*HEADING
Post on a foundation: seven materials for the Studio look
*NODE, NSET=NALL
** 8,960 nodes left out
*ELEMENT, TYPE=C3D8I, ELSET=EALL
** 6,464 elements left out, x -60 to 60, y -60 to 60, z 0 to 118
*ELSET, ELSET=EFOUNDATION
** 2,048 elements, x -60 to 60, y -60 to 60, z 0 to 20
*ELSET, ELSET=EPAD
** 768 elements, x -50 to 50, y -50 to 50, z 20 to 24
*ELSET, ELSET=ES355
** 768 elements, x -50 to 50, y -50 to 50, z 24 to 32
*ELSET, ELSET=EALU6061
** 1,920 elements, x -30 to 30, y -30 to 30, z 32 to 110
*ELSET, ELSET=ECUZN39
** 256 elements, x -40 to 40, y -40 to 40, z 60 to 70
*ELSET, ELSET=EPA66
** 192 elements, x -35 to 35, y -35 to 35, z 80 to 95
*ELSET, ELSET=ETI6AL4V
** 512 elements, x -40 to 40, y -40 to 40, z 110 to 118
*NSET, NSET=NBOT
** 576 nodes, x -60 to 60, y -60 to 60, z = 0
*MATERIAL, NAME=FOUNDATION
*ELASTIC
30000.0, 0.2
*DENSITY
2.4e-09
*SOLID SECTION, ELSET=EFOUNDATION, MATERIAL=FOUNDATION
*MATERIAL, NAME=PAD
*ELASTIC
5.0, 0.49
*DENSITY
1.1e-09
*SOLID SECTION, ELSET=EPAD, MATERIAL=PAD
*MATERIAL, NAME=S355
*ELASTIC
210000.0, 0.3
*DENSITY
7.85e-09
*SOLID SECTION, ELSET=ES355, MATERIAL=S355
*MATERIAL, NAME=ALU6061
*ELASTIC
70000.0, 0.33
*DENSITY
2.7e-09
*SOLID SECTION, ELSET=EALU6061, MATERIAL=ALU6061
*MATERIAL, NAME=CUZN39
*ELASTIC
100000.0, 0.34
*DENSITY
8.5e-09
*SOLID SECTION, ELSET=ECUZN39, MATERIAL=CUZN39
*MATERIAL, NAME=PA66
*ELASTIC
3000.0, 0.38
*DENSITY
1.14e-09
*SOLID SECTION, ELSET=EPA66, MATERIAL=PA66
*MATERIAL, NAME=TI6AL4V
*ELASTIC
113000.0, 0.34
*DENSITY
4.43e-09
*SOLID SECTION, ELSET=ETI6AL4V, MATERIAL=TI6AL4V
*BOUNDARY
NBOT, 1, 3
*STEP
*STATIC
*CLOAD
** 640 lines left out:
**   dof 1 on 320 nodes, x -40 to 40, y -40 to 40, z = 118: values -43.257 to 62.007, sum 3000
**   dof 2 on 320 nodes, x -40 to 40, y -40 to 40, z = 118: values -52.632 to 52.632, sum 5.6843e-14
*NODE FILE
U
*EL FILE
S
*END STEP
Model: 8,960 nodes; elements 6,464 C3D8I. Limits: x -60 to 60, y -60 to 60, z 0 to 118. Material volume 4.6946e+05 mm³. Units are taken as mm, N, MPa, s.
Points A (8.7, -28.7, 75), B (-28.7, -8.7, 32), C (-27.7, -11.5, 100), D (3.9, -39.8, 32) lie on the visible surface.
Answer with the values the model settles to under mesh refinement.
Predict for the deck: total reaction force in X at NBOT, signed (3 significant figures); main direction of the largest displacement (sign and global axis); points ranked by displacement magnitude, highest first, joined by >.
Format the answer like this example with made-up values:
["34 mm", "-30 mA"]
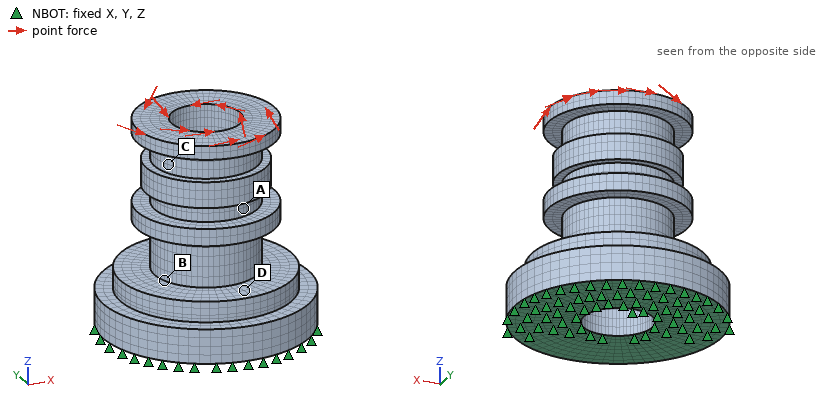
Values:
["-3000 N", "+X", "D > A > C > B"]
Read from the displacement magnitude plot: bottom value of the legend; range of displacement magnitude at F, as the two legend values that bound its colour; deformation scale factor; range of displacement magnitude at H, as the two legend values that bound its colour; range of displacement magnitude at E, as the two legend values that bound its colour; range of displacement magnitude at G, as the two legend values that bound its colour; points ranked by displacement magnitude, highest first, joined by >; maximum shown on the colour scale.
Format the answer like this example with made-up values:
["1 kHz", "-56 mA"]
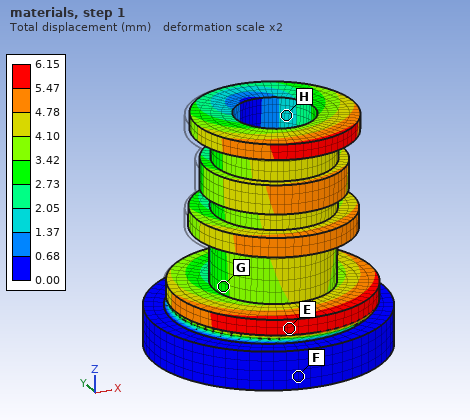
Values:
["0.00 mm", "0.00 to 0.68 mm", "2", "1.37 to 2.05 mm", "5.47 to 6.15 mm", "2.73 to 3.42 mm", "E > G > H > F", "6.15 mm"]
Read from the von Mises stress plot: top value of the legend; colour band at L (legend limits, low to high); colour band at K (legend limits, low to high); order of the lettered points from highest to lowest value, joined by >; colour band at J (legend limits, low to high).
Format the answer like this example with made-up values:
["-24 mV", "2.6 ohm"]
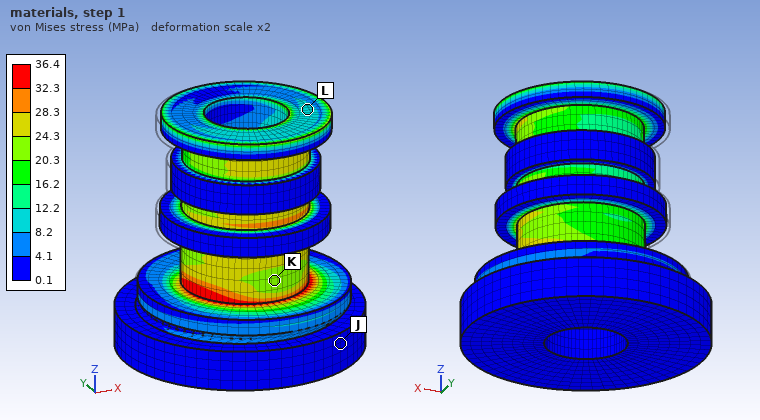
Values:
["36.4 MPa", "8.2 to 12.2 MPa", "20.3 to 24.3 MPa", "K > L > J", "0.1 to 4.1 MPa"]
